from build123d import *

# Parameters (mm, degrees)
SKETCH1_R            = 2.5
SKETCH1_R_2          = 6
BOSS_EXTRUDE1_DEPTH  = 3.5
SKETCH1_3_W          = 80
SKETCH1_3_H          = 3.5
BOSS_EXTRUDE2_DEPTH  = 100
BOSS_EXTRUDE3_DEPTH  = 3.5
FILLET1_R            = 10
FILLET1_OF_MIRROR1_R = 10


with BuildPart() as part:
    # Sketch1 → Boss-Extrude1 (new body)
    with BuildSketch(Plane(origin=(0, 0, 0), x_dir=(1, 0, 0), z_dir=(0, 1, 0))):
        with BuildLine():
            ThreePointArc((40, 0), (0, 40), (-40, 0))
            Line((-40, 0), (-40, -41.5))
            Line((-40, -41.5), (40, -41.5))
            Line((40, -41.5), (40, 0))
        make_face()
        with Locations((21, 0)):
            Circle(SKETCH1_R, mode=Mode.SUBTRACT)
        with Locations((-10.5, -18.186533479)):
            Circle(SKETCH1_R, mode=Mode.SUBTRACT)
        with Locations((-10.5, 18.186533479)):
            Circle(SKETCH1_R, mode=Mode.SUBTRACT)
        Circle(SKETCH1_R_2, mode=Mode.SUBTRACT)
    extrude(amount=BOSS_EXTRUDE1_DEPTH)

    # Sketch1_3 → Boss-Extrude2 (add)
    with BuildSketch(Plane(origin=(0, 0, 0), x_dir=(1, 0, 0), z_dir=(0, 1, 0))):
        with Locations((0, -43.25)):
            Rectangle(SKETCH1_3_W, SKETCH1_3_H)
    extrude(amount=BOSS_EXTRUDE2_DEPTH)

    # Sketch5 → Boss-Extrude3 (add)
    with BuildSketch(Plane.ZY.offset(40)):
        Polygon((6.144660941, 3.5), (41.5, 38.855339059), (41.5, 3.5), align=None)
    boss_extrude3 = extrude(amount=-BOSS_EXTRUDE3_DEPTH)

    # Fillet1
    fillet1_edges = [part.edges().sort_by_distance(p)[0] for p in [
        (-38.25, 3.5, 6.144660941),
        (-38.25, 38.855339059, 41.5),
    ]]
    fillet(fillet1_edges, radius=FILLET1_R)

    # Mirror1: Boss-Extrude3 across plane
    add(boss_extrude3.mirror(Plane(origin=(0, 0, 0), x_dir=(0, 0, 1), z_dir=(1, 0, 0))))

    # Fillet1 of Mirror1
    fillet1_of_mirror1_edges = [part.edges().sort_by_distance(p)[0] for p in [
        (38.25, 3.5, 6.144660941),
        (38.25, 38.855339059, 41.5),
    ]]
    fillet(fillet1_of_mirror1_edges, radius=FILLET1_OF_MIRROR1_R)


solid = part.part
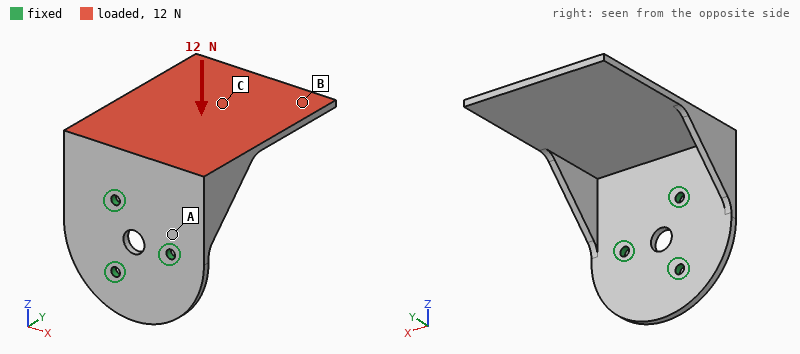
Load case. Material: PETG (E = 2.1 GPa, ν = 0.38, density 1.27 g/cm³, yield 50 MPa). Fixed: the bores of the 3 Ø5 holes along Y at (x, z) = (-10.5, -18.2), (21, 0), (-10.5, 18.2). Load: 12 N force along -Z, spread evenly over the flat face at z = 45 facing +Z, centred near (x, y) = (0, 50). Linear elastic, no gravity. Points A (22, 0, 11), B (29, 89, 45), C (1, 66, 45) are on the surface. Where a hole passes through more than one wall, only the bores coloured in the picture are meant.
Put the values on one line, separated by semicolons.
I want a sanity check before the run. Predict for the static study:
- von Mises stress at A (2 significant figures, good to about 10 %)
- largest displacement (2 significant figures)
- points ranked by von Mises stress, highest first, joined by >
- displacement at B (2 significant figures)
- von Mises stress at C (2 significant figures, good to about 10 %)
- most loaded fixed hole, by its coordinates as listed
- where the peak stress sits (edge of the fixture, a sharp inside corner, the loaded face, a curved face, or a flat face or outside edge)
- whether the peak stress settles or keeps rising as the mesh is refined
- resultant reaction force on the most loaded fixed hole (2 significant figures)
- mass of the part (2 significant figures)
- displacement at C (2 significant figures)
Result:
1.3 MPa; 1.7 mm; A > C > B; 1.5 mm; 0.72 MPa; (-10.5, 18.2); edge of the fixture; keeps rising; 12 N; 66 g; 0.98 mm
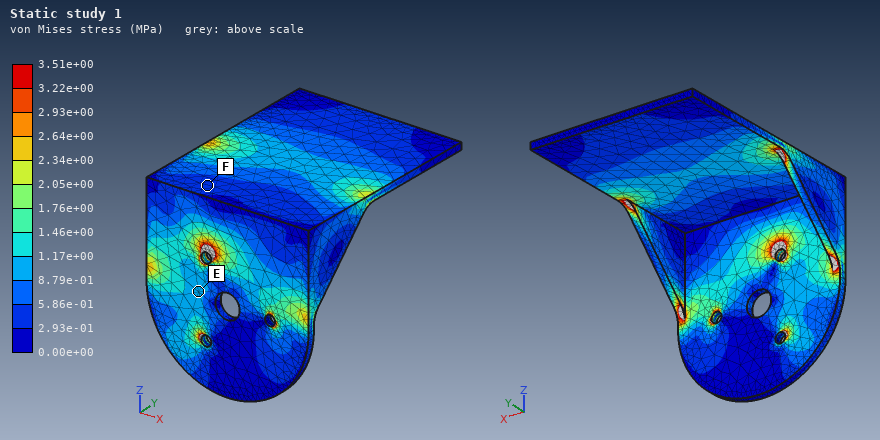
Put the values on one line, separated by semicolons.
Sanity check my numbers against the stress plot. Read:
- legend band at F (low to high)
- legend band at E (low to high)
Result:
2.93e-01 to 5.86e-01 MPa; 8.79e-01 to 1.17e+00 MPa
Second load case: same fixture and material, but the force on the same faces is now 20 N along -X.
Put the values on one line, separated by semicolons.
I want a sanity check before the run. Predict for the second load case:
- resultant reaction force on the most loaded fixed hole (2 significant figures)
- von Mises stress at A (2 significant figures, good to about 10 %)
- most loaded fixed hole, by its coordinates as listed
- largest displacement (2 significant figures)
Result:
27 N; 2.9 MPa; (-10.5, 18.2); 1.7 mm
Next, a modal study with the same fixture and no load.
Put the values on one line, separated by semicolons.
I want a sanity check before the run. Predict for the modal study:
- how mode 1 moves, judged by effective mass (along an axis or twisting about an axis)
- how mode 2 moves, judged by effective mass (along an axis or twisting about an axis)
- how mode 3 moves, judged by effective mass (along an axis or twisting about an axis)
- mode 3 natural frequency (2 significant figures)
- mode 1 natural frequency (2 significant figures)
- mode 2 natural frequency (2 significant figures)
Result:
along Z; along X; along Y; 280 Hz; 84 Hz; 120 Hz
